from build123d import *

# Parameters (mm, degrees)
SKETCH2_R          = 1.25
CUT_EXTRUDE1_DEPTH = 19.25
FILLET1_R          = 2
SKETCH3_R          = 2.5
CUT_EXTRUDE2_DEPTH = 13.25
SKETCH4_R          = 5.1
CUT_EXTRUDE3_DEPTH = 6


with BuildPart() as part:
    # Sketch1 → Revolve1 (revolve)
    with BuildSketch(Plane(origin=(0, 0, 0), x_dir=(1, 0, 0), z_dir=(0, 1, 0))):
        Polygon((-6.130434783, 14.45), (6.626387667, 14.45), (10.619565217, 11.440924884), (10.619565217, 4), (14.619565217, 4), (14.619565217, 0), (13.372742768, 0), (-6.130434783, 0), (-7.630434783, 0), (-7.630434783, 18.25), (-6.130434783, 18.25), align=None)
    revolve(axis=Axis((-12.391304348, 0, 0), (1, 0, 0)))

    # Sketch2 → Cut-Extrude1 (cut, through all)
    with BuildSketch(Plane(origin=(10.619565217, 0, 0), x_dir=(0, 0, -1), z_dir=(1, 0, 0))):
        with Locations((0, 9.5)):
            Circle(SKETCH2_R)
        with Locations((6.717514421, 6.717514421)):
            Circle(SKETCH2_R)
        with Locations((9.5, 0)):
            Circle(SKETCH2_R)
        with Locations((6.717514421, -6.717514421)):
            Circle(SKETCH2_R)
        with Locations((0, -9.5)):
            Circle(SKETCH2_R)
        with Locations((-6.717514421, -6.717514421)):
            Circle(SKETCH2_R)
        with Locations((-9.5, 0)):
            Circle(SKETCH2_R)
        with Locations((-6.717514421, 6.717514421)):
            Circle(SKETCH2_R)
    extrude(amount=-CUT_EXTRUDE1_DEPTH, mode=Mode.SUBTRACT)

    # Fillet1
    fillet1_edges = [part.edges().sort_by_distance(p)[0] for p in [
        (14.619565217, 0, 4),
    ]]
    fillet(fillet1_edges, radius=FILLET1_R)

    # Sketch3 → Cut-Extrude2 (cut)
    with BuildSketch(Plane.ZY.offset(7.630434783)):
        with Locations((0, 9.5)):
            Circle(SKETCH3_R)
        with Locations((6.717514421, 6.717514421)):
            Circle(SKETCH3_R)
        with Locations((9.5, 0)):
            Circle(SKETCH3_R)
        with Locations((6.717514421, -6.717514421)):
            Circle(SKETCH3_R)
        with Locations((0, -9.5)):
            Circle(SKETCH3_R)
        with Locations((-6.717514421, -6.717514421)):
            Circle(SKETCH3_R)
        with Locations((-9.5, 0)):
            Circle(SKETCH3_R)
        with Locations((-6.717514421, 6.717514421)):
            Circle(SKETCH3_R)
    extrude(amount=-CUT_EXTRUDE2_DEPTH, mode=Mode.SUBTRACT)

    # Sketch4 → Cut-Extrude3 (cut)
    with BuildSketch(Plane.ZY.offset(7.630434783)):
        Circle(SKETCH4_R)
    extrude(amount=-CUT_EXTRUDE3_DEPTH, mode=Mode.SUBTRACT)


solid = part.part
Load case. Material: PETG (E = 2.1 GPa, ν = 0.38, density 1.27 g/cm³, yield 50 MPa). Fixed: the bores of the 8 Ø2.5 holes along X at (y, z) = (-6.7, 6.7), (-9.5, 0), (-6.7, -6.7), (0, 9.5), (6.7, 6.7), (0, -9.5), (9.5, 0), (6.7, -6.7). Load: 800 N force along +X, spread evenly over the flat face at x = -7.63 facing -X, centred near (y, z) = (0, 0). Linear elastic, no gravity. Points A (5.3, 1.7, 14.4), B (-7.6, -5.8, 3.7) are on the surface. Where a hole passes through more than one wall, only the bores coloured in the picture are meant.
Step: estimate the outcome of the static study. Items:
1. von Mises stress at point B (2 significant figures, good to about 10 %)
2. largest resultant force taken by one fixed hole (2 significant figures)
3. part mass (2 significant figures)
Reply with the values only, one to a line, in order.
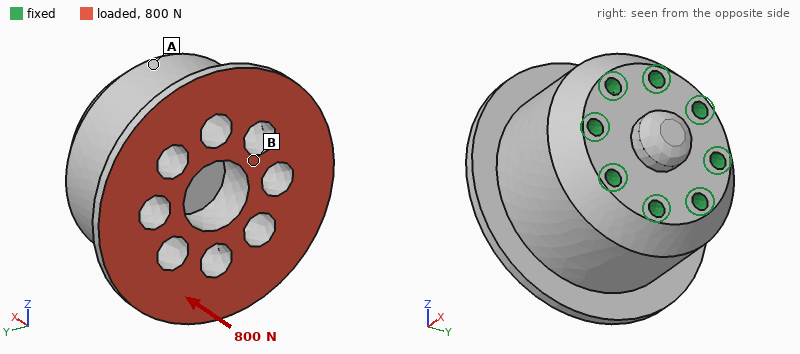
2.9 MPa
100 N
12 g
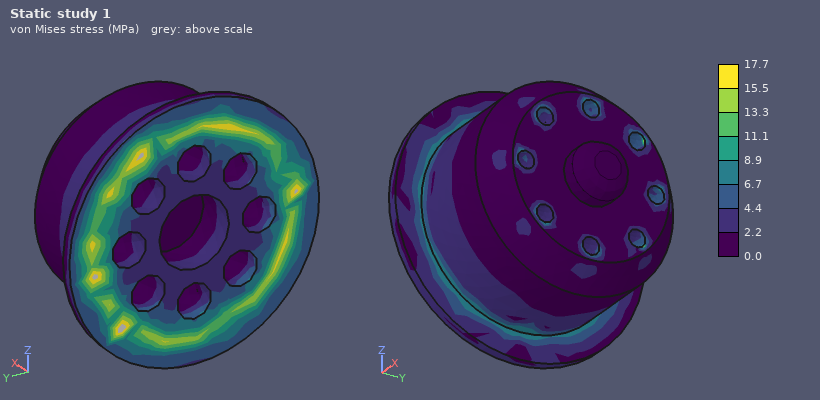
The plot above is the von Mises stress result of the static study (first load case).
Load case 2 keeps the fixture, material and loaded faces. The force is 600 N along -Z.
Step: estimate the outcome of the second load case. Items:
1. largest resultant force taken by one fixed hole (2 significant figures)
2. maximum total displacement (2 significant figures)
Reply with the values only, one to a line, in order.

220 N
0.14 mm
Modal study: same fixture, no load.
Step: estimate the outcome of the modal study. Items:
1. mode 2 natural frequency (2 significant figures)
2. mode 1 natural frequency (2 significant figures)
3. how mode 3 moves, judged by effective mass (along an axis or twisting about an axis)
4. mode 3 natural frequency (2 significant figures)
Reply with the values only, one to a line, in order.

7000 Hz
7000 Hz
twisting about X
9400 Hz
